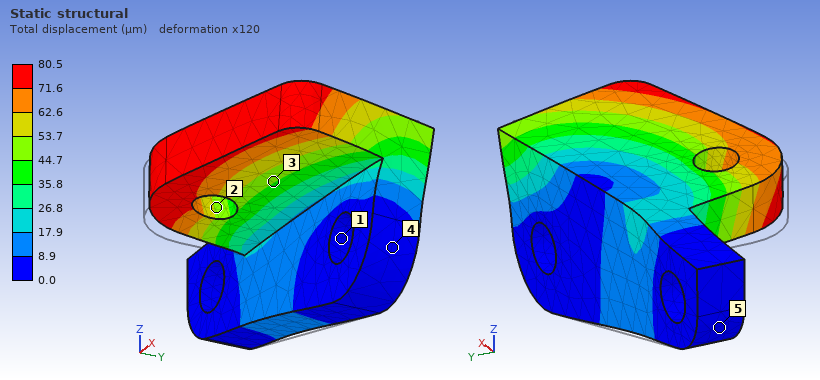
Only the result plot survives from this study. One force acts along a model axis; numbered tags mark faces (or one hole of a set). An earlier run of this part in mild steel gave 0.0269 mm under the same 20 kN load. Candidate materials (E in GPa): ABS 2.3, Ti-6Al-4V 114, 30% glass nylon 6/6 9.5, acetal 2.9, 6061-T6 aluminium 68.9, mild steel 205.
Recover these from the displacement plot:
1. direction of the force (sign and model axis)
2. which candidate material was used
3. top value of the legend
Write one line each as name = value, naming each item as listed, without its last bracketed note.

direction of the force = +X
which candidate material was used = 6061-T6 aluminium
top value of the legend = 80.5 µm
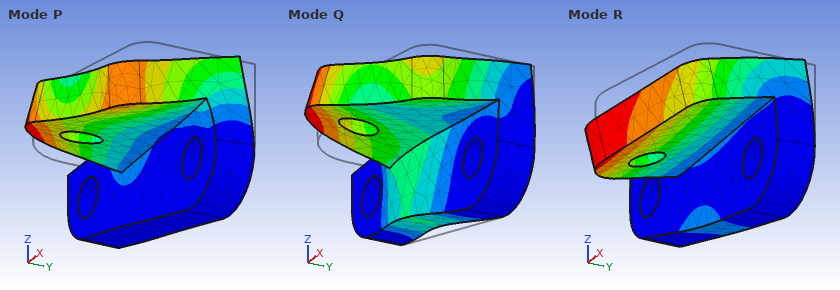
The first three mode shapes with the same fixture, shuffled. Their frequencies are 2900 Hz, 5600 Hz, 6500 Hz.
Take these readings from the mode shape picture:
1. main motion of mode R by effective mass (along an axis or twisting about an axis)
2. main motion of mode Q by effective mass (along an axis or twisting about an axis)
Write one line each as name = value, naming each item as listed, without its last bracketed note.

main motion of mode R by effective mass = along Z
main motion of mode Q by effective mass = along Y
